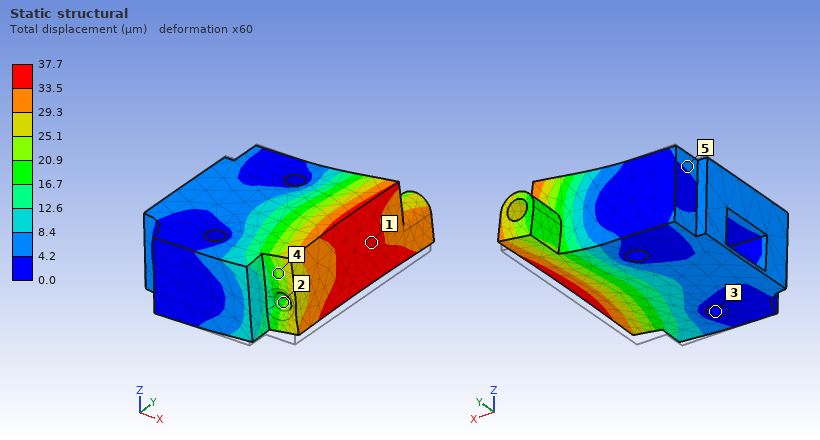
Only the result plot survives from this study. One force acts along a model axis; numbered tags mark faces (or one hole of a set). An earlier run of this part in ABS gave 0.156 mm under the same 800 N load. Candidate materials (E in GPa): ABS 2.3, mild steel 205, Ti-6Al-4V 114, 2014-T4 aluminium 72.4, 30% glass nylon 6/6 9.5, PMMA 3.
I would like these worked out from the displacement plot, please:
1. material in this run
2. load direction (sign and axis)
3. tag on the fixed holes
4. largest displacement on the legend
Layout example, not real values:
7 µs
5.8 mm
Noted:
30% glass nylon 6/6
+Z
3
37.7 µm
